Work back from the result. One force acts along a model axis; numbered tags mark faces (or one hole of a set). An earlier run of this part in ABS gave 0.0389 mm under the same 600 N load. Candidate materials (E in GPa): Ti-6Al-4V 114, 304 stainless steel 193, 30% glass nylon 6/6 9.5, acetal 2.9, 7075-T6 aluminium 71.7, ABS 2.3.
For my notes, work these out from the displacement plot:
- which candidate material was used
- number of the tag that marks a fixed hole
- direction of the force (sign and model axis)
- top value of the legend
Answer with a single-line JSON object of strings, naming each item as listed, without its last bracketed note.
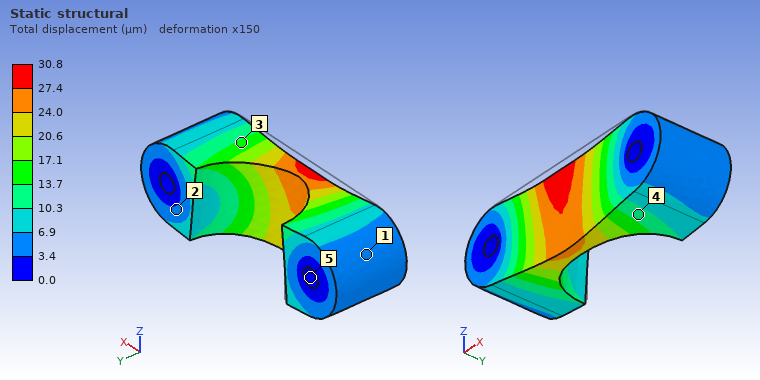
{"which candidate material was used": "acetal", "number of the tag that marks a fixed hole": "5", "direction of the force": "-Z", "top value of the legend": "30.8 µm"}
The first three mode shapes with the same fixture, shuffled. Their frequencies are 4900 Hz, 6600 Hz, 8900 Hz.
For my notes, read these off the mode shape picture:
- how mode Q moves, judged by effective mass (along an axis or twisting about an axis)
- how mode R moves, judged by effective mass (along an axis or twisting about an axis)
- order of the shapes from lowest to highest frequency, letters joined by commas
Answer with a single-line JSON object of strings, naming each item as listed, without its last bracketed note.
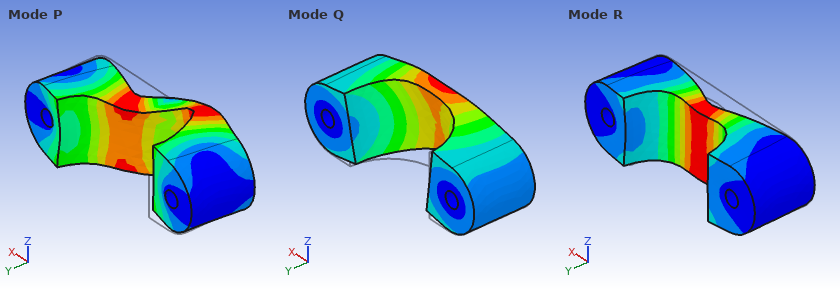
{"how mode Q moves, judged by effective mass": "along Z", "how mode R moves, judged by effective mass": "along Y", "order of the shapes from lowest to highest frequency, letters joined by commas": "Q, R, P"}
